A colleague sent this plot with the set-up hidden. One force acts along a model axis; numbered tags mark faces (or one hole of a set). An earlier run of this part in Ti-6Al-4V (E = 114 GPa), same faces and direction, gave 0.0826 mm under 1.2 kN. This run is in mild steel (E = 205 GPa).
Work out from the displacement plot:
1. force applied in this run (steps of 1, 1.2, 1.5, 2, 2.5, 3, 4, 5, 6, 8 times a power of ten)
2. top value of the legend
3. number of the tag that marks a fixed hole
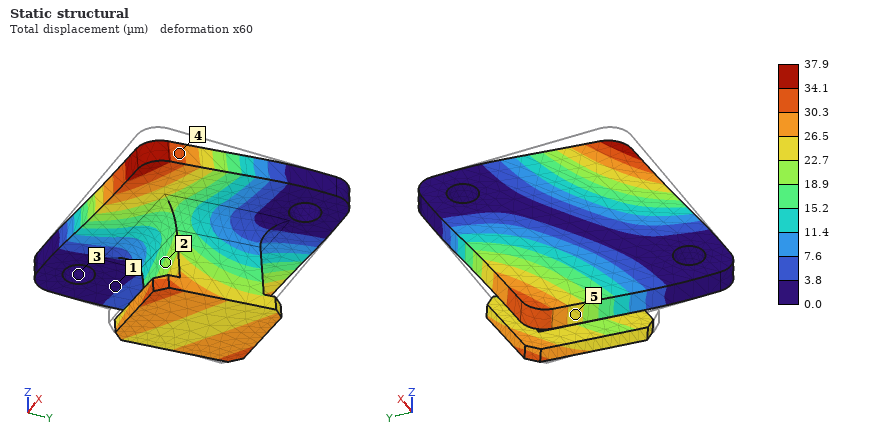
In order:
1 kN
37.9 µm
3
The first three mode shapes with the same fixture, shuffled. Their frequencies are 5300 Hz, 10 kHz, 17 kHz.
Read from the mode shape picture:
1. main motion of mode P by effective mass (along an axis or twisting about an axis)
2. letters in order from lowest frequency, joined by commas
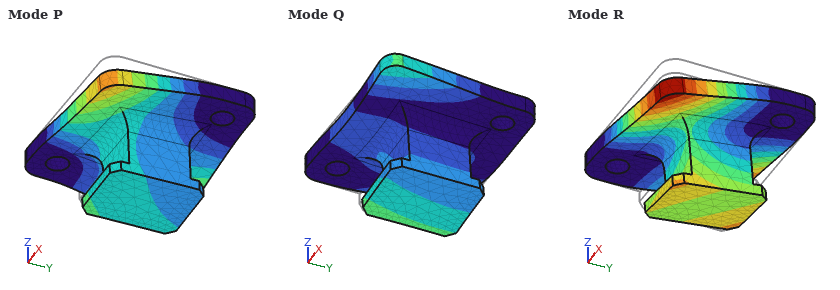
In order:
along Z
R, P, Q
